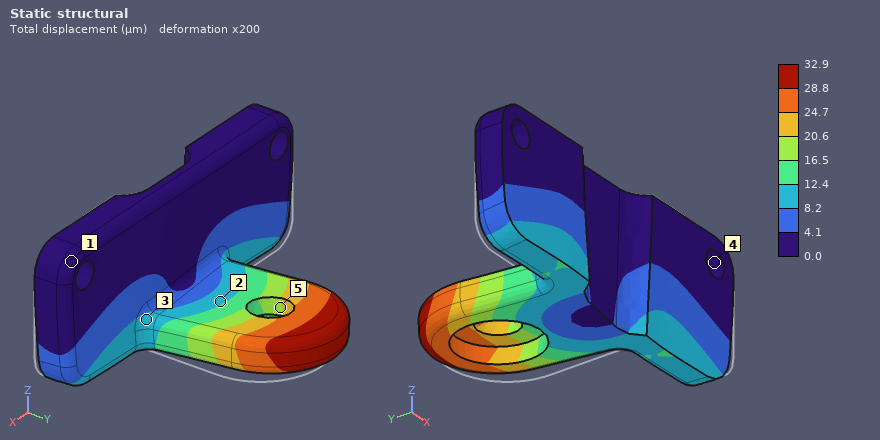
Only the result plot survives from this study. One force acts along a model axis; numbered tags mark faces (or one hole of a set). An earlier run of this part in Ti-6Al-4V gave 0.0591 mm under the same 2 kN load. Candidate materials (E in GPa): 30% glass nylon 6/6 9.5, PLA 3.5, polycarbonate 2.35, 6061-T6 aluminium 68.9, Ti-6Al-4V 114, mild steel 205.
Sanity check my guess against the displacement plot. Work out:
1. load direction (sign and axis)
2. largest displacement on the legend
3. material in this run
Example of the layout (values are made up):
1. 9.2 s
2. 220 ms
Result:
1. -X
2. 32.9 µm
3. mild steel
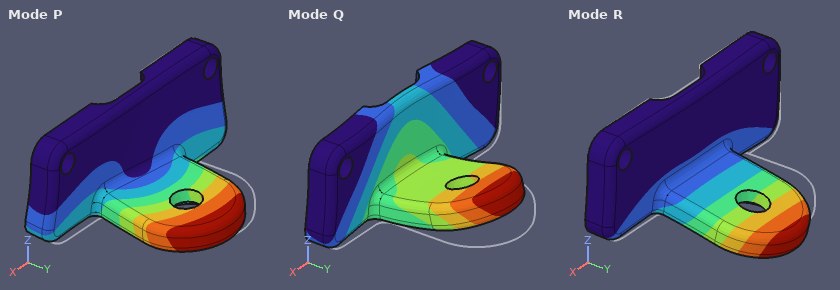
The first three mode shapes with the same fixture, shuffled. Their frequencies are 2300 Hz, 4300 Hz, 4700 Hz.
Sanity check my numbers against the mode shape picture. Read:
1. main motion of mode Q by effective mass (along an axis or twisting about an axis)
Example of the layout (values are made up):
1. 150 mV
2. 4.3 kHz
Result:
1. along Y
